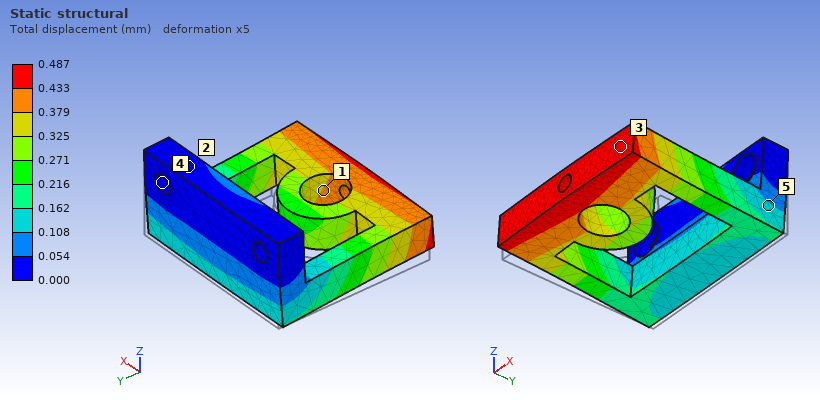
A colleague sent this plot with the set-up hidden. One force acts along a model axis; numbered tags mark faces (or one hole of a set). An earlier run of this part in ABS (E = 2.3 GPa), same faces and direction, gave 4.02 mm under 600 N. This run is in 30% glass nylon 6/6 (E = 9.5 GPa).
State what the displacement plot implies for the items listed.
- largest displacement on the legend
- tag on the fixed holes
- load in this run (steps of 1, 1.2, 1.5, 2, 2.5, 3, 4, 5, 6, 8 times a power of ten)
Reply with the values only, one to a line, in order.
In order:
0.487 mm
4
300 N
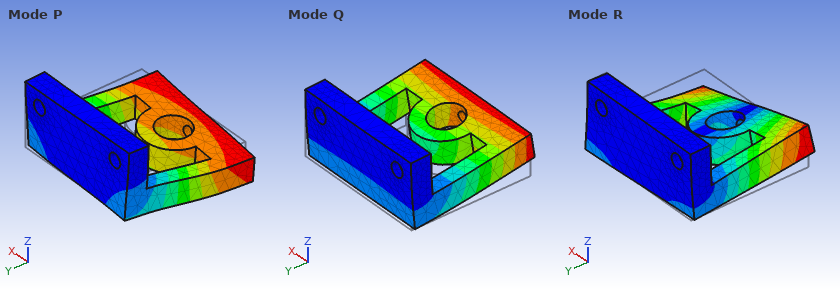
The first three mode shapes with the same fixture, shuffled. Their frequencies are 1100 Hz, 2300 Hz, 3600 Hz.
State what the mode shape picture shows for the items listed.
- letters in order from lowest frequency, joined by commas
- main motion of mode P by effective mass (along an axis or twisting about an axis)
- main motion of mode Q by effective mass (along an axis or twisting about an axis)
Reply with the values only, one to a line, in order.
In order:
Q, P, R
along X
along Z
